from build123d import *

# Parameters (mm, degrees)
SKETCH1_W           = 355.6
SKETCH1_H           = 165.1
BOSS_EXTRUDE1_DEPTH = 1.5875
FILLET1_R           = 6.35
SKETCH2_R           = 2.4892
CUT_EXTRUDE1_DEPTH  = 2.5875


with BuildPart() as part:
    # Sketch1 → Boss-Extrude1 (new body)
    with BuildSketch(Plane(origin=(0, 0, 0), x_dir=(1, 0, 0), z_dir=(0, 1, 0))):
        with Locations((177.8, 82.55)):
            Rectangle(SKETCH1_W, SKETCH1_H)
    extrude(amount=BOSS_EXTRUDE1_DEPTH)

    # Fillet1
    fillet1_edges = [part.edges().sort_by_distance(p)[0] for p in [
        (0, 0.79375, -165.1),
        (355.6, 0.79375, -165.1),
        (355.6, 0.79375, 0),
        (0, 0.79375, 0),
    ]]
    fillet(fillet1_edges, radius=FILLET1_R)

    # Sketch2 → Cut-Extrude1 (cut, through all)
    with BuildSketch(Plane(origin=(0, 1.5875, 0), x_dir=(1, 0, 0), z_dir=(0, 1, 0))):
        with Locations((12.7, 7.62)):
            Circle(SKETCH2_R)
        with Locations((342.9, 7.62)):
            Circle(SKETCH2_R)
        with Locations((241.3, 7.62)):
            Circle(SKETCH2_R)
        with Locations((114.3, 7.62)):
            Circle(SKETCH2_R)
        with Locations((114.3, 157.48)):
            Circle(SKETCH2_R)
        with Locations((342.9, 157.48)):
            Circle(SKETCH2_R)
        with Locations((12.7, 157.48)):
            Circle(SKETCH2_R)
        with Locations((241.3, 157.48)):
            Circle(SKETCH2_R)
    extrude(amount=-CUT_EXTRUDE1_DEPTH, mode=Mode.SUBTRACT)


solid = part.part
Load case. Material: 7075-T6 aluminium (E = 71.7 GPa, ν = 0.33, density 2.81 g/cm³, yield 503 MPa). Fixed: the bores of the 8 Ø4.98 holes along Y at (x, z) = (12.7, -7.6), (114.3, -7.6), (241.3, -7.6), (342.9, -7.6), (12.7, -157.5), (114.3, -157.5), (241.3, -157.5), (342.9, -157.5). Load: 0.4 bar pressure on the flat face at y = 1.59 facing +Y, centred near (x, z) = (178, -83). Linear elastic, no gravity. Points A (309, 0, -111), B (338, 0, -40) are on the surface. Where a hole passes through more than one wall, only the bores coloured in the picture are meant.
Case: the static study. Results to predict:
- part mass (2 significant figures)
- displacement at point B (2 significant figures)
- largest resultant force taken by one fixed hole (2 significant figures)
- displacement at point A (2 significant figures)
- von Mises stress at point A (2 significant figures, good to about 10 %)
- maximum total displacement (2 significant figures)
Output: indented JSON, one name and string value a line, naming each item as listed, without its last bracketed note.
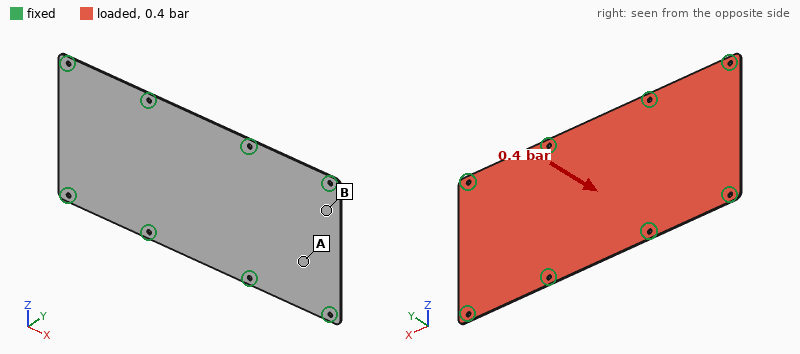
{
  "part mass": "260 g",
  "displacement at point B": "1.5 mm",
  "largest resultant force taken by one fixed hole": "390 N",
  "displacement at point A": "2.6 mm",
  "von Mises stress at point A": "66 MPa",
  "maximum total displacement": "4.4 mm"
}
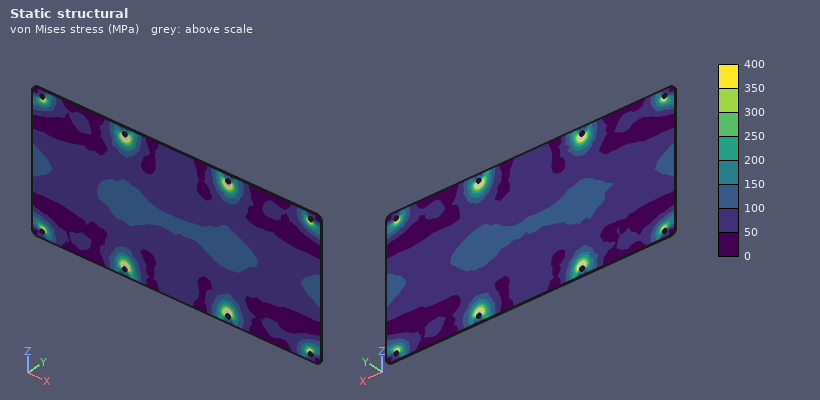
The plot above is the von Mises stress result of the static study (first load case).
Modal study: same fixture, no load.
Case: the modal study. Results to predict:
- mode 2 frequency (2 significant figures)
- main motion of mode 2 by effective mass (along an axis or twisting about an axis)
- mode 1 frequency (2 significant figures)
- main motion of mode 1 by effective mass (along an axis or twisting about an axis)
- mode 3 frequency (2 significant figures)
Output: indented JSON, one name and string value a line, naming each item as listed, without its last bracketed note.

{
  "mode 2 frequency": "320 Hz",
  "main motion of mode 2 by effective mass": "twisting about Z",
  "mode 1 frequency": "280 Hz",
  "main motion of mode 1 by effective mass": "along Y",
  "mode 3 frequency": "350 Hz"
}
